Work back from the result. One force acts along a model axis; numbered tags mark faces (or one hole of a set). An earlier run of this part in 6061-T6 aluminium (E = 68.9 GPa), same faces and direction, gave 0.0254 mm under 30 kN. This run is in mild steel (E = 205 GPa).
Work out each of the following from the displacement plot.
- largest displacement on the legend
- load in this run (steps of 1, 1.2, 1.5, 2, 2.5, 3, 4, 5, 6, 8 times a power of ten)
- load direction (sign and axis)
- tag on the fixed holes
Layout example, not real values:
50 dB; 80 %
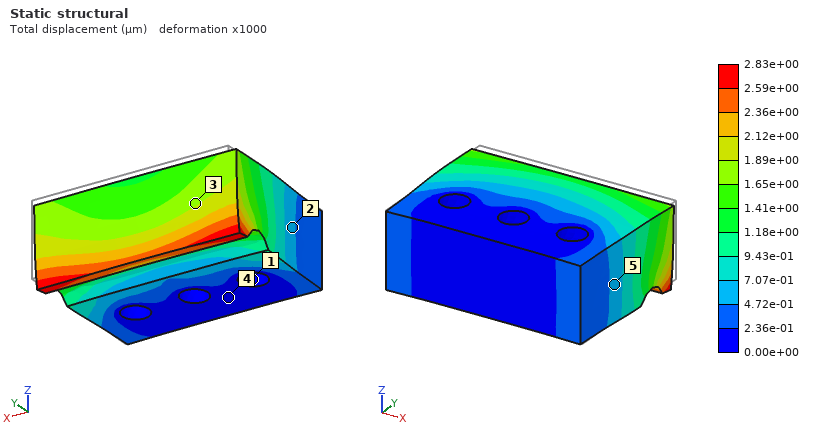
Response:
2.83e+00 µm; 10 kN; -Y; 1
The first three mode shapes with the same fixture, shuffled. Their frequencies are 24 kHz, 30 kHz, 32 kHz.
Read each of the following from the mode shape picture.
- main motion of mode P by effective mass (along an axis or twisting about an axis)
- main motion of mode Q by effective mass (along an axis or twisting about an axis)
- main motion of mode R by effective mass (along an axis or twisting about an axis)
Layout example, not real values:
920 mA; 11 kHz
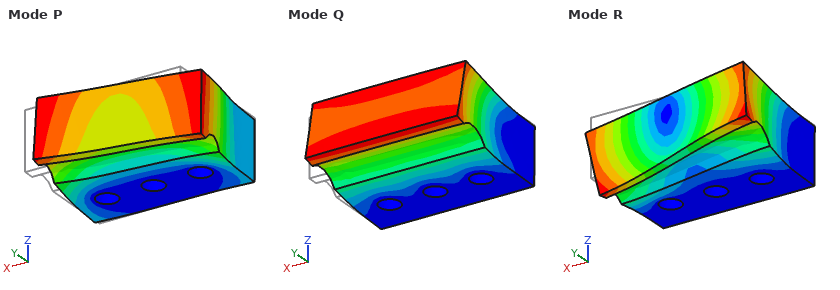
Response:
along X; along Z; twisting about Y
